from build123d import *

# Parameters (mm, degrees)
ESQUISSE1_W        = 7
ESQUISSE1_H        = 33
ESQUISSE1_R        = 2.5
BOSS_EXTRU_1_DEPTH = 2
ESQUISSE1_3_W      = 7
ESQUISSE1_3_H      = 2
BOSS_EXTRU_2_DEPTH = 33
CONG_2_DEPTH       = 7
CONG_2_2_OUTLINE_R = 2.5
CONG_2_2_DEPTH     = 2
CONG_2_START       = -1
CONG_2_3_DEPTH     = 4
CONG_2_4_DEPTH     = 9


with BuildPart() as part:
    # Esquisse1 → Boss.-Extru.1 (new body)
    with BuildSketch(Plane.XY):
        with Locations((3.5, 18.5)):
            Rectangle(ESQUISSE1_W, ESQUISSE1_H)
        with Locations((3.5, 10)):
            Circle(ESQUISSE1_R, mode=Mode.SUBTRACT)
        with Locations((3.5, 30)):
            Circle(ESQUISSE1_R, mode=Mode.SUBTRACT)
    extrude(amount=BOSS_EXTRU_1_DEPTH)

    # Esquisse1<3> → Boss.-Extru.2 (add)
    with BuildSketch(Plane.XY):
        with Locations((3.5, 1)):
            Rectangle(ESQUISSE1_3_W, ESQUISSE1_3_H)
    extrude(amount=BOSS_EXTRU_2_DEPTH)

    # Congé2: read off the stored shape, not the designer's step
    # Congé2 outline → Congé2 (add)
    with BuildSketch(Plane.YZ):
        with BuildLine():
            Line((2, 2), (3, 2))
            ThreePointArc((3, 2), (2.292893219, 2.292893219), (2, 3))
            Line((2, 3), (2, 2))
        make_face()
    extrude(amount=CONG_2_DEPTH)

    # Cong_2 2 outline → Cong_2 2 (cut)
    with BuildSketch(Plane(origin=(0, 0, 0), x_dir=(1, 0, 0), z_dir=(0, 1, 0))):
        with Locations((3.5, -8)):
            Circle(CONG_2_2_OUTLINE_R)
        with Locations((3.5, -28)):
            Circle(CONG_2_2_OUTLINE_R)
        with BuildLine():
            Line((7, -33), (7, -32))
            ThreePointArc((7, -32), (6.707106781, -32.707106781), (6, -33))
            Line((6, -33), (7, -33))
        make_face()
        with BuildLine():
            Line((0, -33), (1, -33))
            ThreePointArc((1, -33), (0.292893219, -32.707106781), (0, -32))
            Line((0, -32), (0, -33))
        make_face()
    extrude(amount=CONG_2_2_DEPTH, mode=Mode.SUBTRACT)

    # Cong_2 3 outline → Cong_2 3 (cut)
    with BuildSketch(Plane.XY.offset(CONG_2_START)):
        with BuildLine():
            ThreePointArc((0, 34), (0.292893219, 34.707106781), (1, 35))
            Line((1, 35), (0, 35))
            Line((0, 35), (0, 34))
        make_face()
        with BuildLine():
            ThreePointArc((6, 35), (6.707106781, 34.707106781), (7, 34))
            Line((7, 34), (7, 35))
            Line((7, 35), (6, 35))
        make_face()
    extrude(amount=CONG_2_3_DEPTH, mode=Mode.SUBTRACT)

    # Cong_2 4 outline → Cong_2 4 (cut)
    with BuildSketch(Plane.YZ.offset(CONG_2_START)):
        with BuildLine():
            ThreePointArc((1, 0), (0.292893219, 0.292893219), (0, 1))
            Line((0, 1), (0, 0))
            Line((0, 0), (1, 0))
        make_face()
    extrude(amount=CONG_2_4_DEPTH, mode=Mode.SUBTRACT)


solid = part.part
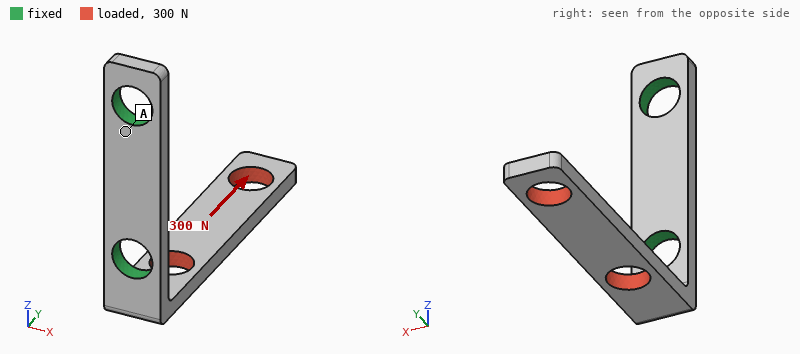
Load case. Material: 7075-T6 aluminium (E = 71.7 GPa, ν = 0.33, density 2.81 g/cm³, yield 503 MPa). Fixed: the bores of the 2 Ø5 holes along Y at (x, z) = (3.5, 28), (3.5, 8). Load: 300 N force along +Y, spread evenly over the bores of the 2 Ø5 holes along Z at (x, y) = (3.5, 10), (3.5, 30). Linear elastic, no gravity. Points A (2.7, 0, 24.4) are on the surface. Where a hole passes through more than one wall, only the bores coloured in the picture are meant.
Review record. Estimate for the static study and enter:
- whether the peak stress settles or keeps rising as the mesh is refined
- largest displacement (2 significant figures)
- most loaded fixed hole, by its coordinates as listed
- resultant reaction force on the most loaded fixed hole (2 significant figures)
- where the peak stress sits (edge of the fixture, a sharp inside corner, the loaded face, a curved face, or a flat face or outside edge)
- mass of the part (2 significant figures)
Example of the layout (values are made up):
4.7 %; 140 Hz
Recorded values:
keeps rising; 0.36 mm; (3.5, 8); 300 N; edge of the fixture; 2.2 g
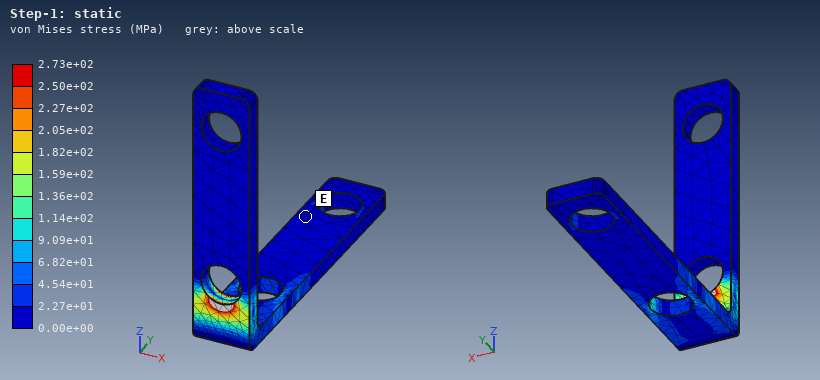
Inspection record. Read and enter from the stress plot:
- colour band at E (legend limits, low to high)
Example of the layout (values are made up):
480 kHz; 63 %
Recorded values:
0.00e+00 to 2.27e+01 MPa
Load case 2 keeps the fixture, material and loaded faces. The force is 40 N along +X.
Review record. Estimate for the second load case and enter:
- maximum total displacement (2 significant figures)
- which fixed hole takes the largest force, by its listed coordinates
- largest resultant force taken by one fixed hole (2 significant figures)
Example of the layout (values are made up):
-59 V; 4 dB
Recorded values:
0.25 mm; (3.5, 8); 40 N
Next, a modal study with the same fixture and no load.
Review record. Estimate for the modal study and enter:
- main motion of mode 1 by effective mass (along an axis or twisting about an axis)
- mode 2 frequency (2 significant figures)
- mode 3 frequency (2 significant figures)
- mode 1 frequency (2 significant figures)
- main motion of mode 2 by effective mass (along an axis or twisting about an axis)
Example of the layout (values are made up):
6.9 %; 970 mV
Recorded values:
along Z; 2500 Hz; 7400 Hz; 1200 Hz; along X
